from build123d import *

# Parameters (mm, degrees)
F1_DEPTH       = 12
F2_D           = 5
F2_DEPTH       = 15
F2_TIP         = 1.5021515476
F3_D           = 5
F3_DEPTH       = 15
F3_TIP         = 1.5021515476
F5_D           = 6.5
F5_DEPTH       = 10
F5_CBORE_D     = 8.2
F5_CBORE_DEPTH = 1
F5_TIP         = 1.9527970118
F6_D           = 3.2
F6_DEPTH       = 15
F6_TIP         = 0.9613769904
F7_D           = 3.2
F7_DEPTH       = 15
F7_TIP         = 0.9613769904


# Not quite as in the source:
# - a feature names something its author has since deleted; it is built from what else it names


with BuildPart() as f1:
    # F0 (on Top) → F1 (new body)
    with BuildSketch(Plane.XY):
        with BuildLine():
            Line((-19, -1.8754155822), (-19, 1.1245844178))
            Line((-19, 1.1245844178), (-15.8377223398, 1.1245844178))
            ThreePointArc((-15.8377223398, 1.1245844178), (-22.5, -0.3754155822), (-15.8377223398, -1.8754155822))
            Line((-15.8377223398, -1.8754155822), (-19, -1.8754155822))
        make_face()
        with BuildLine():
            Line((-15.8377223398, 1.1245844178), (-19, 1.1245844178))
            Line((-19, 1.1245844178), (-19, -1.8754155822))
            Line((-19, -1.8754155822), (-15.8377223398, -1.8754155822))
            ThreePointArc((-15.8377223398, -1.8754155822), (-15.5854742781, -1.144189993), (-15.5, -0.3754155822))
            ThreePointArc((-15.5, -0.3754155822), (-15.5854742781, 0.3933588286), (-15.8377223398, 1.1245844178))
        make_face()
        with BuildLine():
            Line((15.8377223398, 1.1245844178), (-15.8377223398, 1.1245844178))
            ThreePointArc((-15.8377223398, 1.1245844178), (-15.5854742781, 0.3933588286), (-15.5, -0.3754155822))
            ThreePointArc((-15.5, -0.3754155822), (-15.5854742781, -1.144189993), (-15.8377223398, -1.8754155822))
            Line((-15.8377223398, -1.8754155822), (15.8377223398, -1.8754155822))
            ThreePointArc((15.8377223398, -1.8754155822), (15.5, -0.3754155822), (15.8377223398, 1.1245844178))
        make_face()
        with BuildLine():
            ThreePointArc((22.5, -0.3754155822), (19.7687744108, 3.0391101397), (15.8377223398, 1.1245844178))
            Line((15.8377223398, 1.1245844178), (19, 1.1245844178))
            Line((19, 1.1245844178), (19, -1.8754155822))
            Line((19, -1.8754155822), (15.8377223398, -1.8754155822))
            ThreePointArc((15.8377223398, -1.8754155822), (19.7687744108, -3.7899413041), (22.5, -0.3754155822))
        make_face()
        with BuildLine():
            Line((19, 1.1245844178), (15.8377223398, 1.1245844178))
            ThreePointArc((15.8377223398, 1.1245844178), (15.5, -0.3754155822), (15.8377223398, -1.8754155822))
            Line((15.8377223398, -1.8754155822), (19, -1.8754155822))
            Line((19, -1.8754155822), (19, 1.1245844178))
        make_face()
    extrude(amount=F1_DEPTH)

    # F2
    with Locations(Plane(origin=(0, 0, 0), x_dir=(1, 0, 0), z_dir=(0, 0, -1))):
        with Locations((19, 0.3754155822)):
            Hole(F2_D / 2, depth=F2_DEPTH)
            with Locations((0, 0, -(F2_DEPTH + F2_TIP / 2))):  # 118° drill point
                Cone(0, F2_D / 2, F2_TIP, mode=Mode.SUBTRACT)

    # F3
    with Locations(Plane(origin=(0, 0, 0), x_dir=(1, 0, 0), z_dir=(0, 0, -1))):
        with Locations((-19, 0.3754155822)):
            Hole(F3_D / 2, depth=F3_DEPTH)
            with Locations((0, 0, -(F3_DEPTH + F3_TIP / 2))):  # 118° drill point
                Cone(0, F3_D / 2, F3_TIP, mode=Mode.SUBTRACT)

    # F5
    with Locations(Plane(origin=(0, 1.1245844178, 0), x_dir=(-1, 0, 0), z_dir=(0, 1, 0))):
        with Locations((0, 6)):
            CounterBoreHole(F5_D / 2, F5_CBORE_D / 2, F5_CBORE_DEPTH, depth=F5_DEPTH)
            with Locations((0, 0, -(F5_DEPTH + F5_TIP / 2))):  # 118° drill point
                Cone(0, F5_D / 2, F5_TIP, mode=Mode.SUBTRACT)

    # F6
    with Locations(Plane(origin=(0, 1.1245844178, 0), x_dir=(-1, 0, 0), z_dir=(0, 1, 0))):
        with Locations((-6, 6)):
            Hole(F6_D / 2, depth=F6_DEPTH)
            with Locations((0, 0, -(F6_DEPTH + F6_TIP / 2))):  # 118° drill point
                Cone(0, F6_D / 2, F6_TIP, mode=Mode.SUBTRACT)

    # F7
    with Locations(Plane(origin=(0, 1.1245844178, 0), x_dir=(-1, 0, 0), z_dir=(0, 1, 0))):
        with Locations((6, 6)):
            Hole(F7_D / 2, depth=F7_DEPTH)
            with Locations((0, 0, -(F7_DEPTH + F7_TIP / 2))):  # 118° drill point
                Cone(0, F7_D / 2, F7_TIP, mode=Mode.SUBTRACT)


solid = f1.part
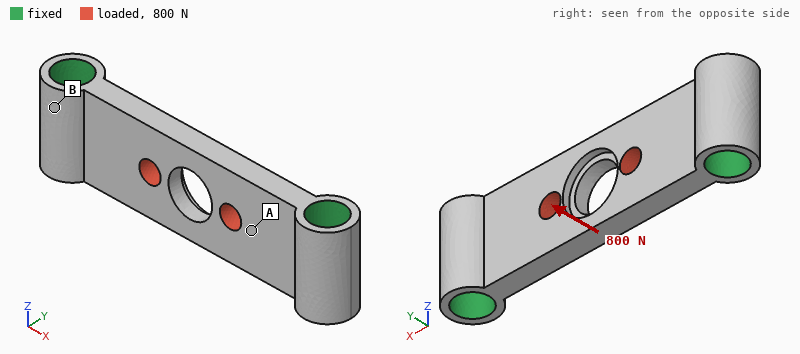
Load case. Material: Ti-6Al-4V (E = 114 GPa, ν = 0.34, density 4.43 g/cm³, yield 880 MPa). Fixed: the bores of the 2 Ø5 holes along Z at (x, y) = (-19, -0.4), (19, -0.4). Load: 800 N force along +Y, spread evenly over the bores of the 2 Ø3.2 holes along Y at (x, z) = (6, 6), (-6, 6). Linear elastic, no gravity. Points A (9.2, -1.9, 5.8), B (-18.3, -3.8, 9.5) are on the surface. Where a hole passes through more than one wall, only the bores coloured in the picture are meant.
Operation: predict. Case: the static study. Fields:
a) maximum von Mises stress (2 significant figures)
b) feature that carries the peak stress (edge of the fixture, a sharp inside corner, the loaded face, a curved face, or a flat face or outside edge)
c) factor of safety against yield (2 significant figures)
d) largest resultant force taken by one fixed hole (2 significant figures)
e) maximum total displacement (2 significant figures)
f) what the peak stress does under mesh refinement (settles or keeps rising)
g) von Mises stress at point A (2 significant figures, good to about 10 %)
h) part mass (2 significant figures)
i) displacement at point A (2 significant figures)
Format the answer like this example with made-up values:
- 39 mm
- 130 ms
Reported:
- 270 MPa
- the loaded face
- 3.2
- 400 N
- 46 µm
- settles
- 42 MPa
- 6.2 g
- 22 µm
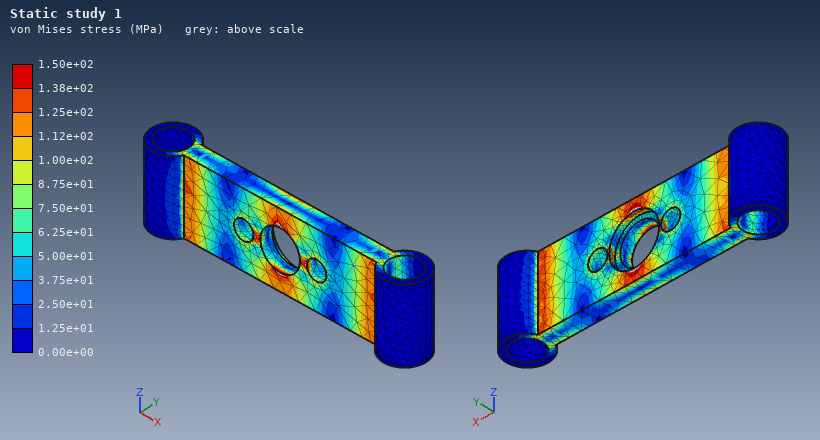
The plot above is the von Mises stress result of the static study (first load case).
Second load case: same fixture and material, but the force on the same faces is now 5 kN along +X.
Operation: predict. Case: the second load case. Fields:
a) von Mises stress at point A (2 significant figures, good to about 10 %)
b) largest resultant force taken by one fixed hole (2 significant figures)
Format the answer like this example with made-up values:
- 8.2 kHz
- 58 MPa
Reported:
- 94 MPa
- 2.5 kN
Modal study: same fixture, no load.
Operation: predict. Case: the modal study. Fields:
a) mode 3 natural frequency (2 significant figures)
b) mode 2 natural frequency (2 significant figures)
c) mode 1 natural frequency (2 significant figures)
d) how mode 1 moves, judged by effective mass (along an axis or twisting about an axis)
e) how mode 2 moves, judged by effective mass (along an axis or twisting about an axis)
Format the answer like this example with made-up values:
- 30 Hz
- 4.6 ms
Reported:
- 35 kHz
- 24 kHz
- 15 kHz
- along Y
- twisting about X
